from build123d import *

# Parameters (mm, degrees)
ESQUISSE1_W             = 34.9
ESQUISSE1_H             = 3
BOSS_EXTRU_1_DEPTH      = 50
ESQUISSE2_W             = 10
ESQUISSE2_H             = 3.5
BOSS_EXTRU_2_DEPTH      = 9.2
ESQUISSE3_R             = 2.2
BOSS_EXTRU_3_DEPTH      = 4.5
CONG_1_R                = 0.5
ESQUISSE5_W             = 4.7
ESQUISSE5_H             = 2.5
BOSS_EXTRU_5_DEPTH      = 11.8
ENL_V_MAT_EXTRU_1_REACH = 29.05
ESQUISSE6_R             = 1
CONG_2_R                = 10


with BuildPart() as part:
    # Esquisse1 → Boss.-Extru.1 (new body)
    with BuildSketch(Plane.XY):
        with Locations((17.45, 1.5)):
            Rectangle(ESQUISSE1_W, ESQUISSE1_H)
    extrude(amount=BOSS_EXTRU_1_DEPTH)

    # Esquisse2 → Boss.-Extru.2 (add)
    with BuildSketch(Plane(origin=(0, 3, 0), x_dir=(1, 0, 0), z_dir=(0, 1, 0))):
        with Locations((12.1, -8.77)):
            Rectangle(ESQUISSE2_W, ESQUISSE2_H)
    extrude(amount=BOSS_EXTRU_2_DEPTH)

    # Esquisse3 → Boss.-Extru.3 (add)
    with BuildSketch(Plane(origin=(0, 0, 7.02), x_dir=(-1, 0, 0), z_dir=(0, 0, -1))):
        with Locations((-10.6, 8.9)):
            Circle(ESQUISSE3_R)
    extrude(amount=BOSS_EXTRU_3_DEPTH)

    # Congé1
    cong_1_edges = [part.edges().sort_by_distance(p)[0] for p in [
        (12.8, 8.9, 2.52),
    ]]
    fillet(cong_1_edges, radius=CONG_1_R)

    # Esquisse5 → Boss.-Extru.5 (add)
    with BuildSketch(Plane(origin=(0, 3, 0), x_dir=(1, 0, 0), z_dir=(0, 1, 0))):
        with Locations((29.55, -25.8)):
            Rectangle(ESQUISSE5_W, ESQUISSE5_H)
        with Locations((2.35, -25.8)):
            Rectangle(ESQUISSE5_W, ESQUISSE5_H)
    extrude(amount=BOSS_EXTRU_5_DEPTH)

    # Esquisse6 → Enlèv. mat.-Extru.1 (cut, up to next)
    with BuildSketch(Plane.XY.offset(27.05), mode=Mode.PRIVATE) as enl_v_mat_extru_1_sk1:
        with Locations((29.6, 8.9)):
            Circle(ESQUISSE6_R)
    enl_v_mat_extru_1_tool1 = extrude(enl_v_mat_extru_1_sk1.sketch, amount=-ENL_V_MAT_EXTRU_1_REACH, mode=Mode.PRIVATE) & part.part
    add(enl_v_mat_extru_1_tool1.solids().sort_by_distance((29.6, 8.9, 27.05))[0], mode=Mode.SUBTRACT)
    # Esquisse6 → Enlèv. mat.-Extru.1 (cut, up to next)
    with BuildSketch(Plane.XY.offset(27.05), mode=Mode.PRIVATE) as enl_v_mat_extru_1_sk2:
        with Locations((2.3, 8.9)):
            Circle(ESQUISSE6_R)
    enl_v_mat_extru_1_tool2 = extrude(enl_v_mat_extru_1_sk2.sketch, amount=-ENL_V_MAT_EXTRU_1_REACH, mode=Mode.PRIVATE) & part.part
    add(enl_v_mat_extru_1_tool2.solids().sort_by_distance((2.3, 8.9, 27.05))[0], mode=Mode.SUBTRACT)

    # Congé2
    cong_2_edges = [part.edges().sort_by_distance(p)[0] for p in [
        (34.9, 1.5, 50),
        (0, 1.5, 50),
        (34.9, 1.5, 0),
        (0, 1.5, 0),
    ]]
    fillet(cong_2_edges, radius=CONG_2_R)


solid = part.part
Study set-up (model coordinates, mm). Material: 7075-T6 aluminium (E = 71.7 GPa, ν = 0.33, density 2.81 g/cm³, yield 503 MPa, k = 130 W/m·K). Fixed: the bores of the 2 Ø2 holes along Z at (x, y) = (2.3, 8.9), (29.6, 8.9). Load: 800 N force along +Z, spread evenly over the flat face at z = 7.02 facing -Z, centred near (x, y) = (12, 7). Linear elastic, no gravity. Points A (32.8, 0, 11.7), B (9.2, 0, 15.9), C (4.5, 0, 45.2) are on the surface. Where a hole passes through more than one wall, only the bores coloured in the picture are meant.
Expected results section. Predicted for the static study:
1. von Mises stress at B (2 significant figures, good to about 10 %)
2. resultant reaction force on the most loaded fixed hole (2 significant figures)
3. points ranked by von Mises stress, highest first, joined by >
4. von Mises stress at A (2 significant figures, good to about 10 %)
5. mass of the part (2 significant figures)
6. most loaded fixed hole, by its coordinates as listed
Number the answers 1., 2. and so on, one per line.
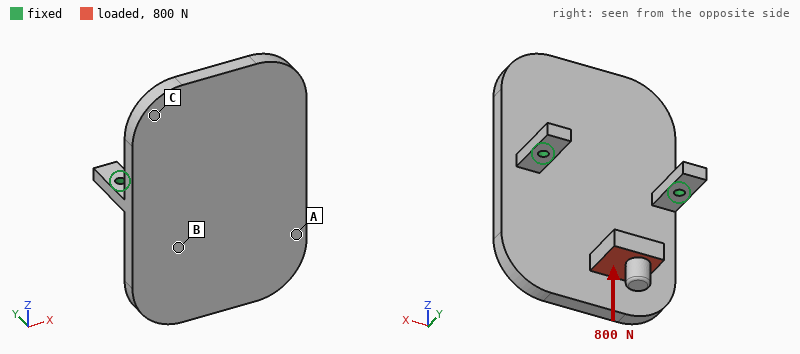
1. 88 MPa
2. 500 N
3. B > A > C
4. 49 MPa
5. 16 g
6. (2.3, 8.9)
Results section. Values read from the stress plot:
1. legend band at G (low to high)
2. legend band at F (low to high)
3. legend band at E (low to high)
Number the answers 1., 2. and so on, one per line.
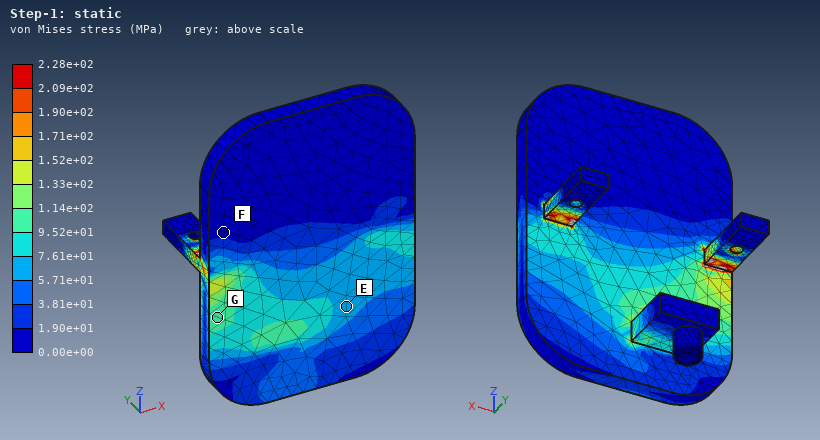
1. 9.52e+01 to 1.14e+02 MPa
2. 0.00e+00 to 1.90e+01 MPa
3. 5.71e+01 to 7.61e+01 MPa
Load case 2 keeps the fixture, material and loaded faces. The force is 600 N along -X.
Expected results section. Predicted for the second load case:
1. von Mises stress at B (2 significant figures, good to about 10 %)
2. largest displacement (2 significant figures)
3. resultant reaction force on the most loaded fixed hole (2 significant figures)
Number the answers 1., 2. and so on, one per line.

1. 52 MPa
2. 0.19 mm
3. 500 N
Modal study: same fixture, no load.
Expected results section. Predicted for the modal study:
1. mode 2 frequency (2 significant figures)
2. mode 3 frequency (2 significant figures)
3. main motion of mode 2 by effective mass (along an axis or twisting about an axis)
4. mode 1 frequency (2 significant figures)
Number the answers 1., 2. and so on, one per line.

1. 3800 Hz
2. 4300 Hz
3. along Y
4. 1000 Hz
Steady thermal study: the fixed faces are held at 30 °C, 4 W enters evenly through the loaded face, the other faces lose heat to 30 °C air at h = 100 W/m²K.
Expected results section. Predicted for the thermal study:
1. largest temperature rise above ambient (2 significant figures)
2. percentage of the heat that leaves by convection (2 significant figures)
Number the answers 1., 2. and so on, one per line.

1. 13 K
2. 55 %
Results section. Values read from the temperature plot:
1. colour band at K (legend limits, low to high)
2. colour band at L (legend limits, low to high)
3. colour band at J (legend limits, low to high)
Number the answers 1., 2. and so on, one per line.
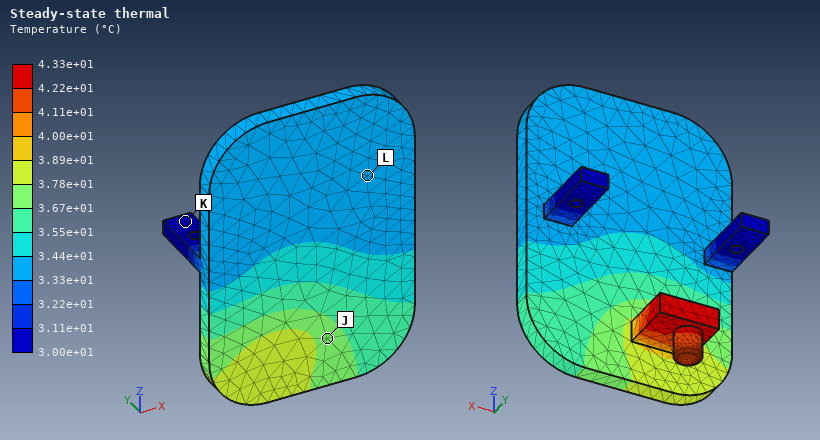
1. 3.00e+01 to 3.11e+01 °C
2. 3.33e+01 to 3.44e+01 °C
3. 3.67e+01 to 3.78e+01 °C
